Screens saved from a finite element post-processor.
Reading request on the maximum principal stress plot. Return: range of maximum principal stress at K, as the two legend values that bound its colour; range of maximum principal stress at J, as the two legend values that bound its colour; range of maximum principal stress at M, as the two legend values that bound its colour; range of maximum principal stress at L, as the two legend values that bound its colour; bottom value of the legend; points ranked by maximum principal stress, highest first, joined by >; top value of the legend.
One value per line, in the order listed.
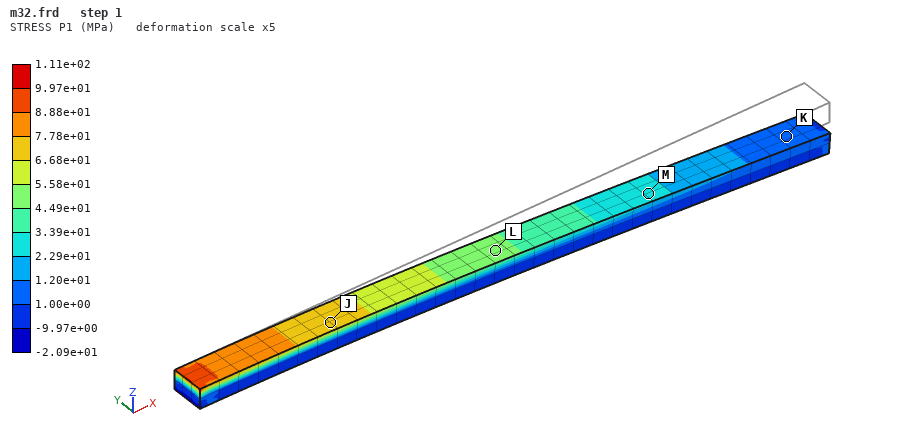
1.00e+00 to 1.20e+01 MPa
6.68e+01 to 7.78e+01 MPa
2.29e+01 to 3.39e+01 MPa
4.49e+01 to 5.58e+01 MPa
-2.09e+01 MPa
J > L > M > K
1.11e+02 MPa
